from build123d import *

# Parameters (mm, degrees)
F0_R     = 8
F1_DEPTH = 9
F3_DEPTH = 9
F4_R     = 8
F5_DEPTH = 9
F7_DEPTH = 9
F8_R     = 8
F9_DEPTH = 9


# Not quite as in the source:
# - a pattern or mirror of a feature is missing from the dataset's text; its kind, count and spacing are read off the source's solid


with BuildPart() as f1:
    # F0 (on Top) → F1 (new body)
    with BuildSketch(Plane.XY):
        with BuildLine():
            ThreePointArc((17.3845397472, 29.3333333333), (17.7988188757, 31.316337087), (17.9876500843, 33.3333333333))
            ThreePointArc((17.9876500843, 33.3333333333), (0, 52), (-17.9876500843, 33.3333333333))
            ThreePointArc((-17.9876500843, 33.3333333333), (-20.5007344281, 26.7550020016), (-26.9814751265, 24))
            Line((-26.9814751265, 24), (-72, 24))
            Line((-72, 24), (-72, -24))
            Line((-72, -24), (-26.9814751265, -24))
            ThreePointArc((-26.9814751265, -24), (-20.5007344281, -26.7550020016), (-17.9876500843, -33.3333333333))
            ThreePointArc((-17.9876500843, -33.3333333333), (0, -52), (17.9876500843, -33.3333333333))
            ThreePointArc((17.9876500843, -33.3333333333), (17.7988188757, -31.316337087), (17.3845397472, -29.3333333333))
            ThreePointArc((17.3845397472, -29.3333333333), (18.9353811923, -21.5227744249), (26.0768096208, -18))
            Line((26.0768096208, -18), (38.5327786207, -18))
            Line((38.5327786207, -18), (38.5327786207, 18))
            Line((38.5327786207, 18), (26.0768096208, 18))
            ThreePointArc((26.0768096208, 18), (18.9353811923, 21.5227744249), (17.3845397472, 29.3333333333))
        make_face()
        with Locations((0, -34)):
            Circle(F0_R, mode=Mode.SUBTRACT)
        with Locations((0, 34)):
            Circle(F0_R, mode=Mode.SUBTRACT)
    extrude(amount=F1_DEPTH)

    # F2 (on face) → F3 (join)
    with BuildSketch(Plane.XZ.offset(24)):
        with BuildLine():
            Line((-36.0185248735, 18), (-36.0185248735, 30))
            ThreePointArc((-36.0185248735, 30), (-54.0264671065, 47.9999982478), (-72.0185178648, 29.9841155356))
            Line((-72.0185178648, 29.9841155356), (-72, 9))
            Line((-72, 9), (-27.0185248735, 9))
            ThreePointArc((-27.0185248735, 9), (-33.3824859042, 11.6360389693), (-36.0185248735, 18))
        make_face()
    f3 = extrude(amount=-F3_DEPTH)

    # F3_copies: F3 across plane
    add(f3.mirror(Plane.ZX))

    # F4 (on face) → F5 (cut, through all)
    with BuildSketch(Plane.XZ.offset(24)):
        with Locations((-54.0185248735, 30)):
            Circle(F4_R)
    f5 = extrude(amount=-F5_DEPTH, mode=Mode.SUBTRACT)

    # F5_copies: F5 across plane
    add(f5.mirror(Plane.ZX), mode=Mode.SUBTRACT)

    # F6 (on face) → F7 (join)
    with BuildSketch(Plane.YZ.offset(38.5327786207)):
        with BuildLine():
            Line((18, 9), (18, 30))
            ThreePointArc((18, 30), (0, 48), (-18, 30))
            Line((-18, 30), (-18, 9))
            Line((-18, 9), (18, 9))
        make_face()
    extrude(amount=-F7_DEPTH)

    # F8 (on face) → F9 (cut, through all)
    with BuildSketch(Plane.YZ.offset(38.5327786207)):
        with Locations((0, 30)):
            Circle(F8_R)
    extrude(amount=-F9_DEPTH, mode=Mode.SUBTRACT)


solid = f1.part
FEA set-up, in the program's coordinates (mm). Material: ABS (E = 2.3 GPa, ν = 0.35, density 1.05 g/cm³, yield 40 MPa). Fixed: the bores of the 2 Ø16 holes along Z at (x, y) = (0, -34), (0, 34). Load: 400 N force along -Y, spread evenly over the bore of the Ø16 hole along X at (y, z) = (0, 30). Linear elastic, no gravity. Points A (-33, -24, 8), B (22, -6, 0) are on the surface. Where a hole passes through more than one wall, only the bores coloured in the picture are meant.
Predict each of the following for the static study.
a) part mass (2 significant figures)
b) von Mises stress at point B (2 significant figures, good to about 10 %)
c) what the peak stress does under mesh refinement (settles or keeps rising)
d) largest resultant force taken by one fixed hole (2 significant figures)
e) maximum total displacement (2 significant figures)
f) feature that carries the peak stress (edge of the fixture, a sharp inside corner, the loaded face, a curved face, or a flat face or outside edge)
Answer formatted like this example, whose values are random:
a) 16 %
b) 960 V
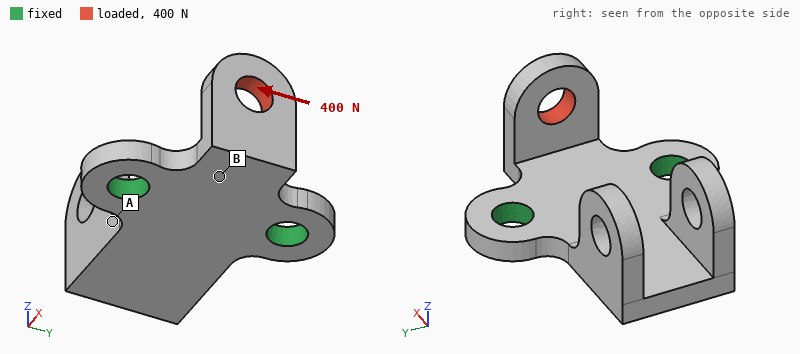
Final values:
a) 91 g
b) 9.1 MPa
c) keeps rising
d) 360 N
e) 1.1 mm
f) a sharp inside corner
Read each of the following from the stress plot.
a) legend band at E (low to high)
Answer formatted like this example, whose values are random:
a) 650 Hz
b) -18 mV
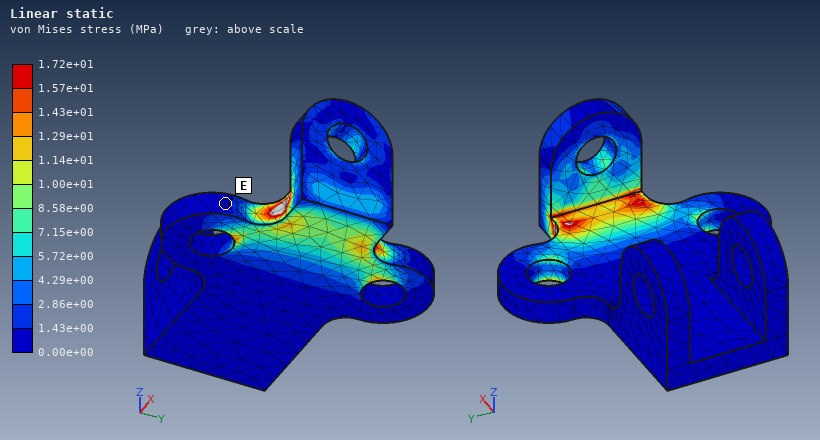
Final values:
a) 0.00e+00 to 1.43e+00 MPa
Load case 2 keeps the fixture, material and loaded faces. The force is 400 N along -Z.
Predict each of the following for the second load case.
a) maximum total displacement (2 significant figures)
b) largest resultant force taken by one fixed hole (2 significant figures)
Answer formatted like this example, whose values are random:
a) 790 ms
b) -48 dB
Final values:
a) 1.9 mm
b) 200 N
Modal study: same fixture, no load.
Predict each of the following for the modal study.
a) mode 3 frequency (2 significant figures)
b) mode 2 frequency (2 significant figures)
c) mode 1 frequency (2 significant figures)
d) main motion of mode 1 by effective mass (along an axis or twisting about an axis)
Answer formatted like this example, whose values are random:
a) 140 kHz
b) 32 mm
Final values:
a) 630 Hz
b) 600 Hz
c) 290 Hz
d) along Z
